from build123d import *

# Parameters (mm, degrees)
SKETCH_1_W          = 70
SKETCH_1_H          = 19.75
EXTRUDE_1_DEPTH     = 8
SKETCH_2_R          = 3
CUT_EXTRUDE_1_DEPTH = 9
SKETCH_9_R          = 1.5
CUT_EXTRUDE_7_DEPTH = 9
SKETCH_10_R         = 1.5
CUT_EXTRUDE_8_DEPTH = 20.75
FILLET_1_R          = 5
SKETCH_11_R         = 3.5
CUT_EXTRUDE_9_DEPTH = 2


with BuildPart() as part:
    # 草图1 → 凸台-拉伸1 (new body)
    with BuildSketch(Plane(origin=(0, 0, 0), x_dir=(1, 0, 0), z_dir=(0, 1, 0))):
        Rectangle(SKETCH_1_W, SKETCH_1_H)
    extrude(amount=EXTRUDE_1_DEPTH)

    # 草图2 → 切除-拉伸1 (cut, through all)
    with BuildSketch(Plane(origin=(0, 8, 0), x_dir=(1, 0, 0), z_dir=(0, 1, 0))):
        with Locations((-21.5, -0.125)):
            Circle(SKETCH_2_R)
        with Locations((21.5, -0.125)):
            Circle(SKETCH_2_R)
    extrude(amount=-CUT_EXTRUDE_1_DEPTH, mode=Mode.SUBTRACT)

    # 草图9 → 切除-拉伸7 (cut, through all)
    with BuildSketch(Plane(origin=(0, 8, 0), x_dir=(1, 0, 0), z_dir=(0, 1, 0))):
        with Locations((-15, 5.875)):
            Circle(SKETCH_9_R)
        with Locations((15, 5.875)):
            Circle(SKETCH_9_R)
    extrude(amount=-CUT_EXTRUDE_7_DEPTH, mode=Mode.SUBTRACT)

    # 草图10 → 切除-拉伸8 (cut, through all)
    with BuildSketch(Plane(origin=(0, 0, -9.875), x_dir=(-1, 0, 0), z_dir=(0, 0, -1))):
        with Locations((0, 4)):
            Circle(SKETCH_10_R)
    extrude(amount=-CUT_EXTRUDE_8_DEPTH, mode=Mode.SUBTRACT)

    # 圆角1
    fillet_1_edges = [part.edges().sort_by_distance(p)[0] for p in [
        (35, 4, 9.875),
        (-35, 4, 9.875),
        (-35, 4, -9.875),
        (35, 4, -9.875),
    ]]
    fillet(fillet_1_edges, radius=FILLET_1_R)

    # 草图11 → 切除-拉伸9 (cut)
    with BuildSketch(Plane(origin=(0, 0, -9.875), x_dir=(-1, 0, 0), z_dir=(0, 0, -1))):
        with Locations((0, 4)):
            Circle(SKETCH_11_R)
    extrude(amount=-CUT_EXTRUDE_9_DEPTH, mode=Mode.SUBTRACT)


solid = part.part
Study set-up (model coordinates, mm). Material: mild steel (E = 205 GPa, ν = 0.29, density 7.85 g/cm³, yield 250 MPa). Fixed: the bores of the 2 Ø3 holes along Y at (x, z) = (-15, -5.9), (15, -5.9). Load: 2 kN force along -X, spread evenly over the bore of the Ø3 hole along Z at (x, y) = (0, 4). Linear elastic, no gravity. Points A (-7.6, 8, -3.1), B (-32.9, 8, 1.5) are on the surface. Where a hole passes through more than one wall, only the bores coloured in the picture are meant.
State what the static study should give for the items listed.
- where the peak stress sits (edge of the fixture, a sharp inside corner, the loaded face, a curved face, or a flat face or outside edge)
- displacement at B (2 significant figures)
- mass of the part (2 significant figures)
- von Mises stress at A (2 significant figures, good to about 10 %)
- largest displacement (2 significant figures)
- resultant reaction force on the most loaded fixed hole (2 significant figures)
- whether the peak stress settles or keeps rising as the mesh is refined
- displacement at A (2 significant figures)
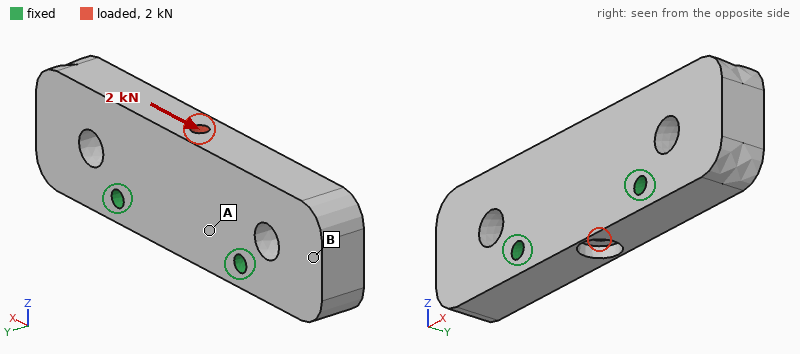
edge of the fixture
1.3 µm
79 g
12 MPa
1.6 µm
1.1 kN
keeps rising
0.53 µm
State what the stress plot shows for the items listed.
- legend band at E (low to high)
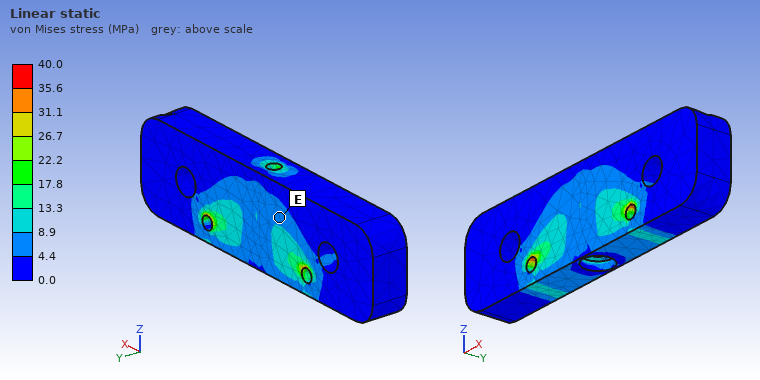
4.4 to 8.9 MPa
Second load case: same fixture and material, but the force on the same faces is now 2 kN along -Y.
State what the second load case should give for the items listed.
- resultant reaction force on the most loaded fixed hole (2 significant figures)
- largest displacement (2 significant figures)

1.0 kN
10 µm
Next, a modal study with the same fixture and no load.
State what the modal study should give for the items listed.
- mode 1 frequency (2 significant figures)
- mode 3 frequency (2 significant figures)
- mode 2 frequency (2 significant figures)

11 kHz
15 kHz
11 kHz
